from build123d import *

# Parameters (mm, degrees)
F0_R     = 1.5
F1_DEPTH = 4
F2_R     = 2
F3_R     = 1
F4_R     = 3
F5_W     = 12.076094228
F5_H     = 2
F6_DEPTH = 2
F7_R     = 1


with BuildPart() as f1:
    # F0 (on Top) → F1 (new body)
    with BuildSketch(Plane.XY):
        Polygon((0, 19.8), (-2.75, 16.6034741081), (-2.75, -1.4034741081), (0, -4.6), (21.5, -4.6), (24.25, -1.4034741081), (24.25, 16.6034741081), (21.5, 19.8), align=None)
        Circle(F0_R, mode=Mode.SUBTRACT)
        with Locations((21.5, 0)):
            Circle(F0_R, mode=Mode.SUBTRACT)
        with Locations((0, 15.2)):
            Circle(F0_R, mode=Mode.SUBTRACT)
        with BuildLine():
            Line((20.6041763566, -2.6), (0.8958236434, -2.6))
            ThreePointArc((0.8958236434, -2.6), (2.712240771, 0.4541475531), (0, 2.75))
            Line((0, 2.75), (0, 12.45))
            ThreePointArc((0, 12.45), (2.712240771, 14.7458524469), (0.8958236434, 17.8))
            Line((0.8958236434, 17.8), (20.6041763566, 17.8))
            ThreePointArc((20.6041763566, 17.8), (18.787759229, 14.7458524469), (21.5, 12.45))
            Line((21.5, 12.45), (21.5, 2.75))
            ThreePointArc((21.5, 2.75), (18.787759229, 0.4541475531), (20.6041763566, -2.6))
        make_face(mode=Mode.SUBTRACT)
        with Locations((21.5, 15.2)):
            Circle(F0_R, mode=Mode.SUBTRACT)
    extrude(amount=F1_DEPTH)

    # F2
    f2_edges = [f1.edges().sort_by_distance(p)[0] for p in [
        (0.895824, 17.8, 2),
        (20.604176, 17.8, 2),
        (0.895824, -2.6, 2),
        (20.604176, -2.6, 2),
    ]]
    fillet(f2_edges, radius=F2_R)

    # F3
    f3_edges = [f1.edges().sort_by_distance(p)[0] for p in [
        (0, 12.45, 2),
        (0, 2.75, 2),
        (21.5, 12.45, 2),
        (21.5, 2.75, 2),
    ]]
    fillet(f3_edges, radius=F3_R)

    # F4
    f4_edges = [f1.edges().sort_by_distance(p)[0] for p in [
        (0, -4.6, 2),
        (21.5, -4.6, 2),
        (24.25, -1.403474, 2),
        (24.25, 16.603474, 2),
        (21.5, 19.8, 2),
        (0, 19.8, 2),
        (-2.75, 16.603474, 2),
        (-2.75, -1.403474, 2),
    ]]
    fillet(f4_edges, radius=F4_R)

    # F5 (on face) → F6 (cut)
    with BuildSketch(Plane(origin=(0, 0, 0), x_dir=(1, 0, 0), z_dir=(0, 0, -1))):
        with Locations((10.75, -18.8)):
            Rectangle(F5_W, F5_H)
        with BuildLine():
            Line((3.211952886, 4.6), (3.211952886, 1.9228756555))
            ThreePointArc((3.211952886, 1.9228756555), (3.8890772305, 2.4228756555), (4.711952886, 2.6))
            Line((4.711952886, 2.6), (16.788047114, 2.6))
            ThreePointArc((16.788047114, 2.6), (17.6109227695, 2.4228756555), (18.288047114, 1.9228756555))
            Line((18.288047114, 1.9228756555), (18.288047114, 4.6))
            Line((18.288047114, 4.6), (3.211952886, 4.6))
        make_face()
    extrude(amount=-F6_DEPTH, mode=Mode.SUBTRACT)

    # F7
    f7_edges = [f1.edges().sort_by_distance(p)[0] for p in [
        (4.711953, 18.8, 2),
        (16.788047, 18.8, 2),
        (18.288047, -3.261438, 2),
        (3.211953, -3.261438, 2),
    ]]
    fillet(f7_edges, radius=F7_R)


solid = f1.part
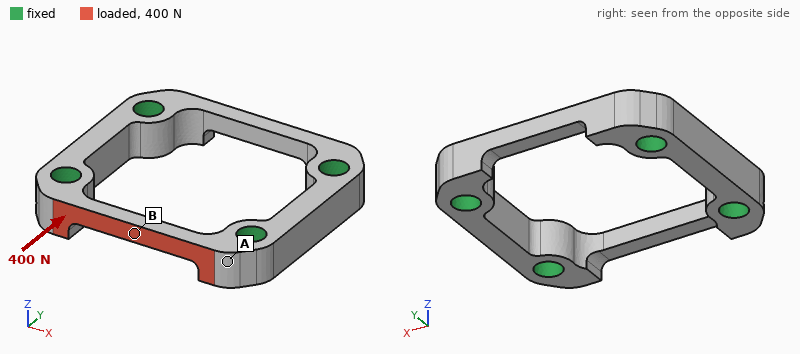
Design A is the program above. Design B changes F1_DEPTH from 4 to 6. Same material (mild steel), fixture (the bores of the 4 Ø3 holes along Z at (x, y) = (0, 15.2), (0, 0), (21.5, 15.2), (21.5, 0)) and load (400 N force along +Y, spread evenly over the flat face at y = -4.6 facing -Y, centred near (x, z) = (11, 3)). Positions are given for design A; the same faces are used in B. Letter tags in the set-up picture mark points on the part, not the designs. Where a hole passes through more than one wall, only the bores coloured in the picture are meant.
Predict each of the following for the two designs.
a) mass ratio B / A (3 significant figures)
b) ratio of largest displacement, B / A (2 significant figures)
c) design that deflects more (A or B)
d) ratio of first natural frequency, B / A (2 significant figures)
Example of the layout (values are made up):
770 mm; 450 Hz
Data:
1.57; 0.58; A; 1.0
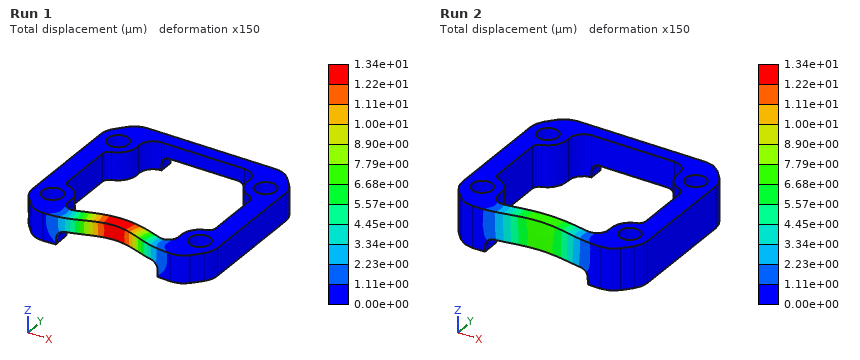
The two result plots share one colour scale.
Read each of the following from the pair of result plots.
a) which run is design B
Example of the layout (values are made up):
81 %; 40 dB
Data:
Run 2
